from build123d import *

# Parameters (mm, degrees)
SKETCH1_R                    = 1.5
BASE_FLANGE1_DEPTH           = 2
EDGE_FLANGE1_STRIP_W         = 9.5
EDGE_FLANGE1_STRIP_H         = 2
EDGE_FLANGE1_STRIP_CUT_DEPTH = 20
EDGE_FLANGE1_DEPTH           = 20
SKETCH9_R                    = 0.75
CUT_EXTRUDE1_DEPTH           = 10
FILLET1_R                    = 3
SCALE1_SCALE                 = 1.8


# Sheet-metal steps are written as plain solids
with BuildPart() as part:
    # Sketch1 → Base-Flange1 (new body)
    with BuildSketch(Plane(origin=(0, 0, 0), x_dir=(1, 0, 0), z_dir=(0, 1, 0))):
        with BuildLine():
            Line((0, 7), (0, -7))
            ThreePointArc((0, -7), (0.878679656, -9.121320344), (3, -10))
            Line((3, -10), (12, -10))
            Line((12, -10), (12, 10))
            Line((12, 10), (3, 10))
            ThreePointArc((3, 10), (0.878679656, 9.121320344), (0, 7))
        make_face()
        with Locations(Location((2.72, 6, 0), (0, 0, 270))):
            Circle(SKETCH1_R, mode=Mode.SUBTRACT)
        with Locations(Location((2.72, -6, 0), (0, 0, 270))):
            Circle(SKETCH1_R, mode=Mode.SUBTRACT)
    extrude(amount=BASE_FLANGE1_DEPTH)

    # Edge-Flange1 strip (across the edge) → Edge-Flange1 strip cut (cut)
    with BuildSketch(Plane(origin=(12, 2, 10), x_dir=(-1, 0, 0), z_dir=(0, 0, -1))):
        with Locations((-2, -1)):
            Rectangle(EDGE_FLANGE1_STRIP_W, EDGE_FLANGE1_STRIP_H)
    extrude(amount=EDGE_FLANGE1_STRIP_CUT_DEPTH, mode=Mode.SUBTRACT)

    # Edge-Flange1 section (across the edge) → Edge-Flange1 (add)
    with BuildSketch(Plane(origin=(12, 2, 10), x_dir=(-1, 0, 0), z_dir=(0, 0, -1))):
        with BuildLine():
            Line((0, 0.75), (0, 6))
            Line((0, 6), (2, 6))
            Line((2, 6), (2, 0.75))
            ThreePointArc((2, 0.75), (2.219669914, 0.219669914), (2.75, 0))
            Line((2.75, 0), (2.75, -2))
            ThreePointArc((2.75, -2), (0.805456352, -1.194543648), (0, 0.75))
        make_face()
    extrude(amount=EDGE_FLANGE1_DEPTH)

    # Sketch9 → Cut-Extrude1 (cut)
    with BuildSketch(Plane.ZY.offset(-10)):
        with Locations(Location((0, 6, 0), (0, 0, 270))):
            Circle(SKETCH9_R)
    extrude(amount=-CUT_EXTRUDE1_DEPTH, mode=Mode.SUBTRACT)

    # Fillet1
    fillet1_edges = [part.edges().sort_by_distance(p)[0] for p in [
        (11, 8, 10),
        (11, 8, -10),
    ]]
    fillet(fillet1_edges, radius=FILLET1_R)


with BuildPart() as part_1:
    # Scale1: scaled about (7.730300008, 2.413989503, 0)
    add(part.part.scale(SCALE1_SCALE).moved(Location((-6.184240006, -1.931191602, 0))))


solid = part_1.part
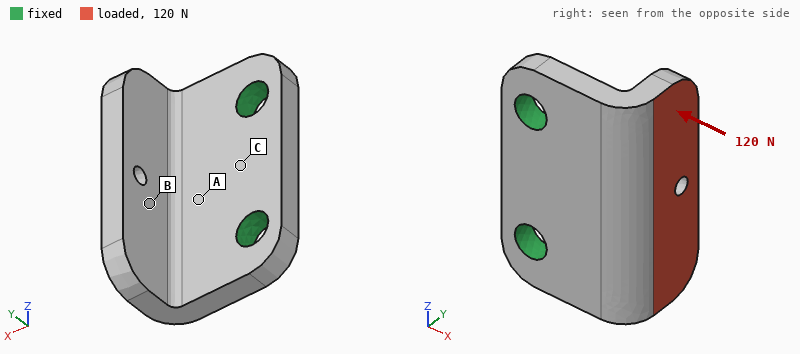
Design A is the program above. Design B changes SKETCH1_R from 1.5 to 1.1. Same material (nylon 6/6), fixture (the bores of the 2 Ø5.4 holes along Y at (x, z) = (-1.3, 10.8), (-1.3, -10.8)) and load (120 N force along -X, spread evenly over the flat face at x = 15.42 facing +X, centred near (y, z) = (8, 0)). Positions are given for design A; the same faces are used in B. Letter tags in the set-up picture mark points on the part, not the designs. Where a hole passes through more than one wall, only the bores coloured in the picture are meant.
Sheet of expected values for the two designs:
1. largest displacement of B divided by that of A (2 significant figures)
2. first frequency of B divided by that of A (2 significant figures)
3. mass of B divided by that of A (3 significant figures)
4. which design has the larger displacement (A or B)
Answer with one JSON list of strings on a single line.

["1.1", "0.91", "1.02", "B"]
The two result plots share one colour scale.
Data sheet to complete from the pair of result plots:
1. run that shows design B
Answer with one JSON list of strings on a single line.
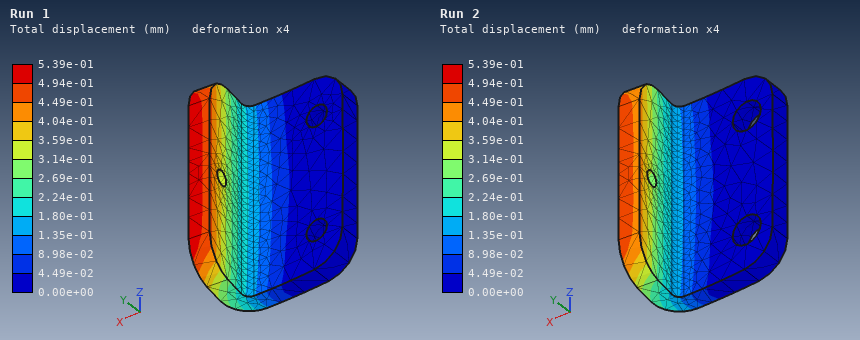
["Run 1"]
